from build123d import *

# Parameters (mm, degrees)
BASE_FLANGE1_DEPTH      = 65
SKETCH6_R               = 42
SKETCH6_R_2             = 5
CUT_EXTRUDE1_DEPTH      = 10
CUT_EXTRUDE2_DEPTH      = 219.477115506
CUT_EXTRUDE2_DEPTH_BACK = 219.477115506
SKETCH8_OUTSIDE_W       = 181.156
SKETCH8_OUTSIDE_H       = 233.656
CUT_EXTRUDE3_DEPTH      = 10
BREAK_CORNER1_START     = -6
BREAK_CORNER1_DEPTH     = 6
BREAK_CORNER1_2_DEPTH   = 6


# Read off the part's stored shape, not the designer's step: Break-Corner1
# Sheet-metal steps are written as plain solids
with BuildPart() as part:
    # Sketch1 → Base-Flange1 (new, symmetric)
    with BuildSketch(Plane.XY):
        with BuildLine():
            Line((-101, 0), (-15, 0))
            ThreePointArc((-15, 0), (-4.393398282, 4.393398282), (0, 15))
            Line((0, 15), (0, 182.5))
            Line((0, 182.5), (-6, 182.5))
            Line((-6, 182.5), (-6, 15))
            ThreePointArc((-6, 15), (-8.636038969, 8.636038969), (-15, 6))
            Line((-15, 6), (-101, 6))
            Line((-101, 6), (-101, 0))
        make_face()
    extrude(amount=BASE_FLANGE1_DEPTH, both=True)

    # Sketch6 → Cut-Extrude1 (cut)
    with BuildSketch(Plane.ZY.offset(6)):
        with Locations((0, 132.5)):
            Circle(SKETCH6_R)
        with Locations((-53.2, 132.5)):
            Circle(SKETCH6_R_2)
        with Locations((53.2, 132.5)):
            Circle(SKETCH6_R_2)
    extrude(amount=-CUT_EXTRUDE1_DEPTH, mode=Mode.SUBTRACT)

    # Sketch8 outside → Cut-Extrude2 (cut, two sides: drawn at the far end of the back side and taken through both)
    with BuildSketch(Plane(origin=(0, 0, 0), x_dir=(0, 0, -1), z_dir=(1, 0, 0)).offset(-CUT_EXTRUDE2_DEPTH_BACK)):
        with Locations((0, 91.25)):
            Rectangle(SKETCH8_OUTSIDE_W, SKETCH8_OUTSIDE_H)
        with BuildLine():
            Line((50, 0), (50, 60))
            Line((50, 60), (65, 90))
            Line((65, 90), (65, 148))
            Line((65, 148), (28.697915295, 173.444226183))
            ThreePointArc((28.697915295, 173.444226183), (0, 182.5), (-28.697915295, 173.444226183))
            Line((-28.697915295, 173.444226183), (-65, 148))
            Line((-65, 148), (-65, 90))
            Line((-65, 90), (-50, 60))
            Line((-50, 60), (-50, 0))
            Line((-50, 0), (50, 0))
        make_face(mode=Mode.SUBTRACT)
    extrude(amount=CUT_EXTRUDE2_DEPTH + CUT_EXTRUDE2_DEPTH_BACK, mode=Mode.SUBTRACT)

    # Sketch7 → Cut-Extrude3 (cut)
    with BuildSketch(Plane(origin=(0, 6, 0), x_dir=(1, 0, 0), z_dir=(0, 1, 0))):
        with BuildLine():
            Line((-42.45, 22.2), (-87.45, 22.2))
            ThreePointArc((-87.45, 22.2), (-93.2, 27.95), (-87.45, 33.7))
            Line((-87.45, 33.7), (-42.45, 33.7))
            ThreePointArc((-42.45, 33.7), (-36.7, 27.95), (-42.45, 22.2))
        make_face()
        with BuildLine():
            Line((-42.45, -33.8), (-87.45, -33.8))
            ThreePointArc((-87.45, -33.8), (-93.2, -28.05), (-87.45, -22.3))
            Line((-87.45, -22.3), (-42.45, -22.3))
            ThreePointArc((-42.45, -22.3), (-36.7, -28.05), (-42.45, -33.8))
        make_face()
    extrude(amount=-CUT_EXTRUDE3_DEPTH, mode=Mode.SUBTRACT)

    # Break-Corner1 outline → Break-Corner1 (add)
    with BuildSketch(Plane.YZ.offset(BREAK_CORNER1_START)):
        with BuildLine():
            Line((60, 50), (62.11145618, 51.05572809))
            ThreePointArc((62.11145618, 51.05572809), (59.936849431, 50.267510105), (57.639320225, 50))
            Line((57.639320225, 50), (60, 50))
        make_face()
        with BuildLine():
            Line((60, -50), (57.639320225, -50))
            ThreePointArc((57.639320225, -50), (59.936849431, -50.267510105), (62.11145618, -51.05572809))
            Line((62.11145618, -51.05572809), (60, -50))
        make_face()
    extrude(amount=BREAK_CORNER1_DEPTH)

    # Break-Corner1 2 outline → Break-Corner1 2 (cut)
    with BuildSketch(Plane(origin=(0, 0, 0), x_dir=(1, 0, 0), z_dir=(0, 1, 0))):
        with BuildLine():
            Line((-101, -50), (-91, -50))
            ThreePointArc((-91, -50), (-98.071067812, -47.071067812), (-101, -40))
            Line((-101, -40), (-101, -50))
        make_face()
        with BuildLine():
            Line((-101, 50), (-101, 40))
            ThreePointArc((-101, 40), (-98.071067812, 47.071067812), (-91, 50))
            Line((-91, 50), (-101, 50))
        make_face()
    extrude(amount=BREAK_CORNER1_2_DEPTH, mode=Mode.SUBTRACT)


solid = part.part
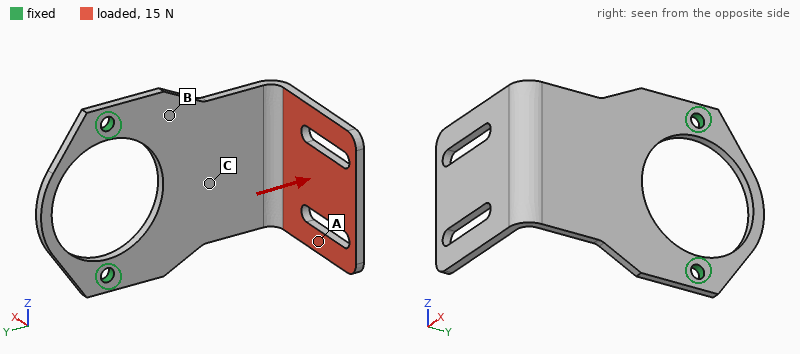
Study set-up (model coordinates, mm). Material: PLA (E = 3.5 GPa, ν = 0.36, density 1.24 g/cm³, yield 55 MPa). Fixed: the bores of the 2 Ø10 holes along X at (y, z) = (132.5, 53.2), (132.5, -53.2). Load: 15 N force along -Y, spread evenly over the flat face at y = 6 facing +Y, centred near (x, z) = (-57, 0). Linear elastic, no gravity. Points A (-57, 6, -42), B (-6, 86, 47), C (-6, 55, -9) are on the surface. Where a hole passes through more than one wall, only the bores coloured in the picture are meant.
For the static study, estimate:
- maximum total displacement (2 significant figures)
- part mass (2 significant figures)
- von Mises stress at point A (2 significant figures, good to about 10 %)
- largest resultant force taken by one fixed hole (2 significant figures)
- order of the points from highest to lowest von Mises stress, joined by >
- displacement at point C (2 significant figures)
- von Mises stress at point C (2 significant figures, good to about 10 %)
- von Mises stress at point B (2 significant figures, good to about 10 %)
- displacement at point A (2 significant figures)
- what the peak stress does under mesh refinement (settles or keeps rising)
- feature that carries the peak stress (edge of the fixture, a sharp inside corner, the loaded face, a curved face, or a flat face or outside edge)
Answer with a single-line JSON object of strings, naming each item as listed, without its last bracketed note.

{"maximum total displacement": "2.7 mm", "part mass": "160 g", "von Mises stress at point A": "0.36 MPa", "largest resultant force taken by one fixed hole": "7.9 N", "order of the points from highest to lowest von Mises stress, joined by >": "B > C > A", "displacement at point C": "0.60 mm", "von Mises stress at point C": "1.1 MPa", "von Mises stress at point B": "1.6 MPa", "displacement at point A": "1.8 mm", "what the peak stress does under mesh refinement": "keeps rising", "feature that carries the peak stress": "edge of the fixture"}
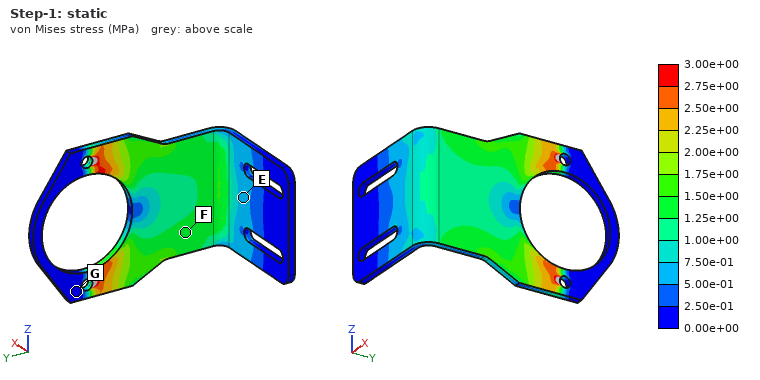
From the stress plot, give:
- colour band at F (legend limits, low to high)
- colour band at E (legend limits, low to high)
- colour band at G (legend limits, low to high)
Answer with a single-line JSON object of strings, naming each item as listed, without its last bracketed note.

{"colour band at F": "1.25e+00 to 1.50e+00 MPa", "colour band at E": "5.00e-01 to 7.50e-01 MPa", "colour band at G": "0.00e+00 to 2.50e-01 MPa"}
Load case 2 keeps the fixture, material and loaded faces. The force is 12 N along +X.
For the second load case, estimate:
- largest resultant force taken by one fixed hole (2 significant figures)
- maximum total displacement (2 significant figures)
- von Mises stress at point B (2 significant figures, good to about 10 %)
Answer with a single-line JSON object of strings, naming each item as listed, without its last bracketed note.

{"largest resultant force taken by one fixed hole": "6.0 N", "maximum total displacement": "2.9 mm", "von Mises stress at point B": "2.0 MPa"}
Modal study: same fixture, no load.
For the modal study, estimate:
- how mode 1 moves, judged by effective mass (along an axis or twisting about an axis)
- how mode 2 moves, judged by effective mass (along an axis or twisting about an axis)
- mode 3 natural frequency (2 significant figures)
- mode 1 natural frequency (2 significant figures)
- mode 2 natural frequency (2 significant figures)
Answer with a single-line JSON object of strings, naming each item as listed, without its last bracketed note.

{"how mode 1 moves, judged by effective mass": "along X", "how mode 2 moves, judged by effective mass": "along Z", "mode 3 natural frequency": "140 Hz", "mode 1 natural frequency": "37 Hz", "mode 2 natural frequency": "98 Hz"}
